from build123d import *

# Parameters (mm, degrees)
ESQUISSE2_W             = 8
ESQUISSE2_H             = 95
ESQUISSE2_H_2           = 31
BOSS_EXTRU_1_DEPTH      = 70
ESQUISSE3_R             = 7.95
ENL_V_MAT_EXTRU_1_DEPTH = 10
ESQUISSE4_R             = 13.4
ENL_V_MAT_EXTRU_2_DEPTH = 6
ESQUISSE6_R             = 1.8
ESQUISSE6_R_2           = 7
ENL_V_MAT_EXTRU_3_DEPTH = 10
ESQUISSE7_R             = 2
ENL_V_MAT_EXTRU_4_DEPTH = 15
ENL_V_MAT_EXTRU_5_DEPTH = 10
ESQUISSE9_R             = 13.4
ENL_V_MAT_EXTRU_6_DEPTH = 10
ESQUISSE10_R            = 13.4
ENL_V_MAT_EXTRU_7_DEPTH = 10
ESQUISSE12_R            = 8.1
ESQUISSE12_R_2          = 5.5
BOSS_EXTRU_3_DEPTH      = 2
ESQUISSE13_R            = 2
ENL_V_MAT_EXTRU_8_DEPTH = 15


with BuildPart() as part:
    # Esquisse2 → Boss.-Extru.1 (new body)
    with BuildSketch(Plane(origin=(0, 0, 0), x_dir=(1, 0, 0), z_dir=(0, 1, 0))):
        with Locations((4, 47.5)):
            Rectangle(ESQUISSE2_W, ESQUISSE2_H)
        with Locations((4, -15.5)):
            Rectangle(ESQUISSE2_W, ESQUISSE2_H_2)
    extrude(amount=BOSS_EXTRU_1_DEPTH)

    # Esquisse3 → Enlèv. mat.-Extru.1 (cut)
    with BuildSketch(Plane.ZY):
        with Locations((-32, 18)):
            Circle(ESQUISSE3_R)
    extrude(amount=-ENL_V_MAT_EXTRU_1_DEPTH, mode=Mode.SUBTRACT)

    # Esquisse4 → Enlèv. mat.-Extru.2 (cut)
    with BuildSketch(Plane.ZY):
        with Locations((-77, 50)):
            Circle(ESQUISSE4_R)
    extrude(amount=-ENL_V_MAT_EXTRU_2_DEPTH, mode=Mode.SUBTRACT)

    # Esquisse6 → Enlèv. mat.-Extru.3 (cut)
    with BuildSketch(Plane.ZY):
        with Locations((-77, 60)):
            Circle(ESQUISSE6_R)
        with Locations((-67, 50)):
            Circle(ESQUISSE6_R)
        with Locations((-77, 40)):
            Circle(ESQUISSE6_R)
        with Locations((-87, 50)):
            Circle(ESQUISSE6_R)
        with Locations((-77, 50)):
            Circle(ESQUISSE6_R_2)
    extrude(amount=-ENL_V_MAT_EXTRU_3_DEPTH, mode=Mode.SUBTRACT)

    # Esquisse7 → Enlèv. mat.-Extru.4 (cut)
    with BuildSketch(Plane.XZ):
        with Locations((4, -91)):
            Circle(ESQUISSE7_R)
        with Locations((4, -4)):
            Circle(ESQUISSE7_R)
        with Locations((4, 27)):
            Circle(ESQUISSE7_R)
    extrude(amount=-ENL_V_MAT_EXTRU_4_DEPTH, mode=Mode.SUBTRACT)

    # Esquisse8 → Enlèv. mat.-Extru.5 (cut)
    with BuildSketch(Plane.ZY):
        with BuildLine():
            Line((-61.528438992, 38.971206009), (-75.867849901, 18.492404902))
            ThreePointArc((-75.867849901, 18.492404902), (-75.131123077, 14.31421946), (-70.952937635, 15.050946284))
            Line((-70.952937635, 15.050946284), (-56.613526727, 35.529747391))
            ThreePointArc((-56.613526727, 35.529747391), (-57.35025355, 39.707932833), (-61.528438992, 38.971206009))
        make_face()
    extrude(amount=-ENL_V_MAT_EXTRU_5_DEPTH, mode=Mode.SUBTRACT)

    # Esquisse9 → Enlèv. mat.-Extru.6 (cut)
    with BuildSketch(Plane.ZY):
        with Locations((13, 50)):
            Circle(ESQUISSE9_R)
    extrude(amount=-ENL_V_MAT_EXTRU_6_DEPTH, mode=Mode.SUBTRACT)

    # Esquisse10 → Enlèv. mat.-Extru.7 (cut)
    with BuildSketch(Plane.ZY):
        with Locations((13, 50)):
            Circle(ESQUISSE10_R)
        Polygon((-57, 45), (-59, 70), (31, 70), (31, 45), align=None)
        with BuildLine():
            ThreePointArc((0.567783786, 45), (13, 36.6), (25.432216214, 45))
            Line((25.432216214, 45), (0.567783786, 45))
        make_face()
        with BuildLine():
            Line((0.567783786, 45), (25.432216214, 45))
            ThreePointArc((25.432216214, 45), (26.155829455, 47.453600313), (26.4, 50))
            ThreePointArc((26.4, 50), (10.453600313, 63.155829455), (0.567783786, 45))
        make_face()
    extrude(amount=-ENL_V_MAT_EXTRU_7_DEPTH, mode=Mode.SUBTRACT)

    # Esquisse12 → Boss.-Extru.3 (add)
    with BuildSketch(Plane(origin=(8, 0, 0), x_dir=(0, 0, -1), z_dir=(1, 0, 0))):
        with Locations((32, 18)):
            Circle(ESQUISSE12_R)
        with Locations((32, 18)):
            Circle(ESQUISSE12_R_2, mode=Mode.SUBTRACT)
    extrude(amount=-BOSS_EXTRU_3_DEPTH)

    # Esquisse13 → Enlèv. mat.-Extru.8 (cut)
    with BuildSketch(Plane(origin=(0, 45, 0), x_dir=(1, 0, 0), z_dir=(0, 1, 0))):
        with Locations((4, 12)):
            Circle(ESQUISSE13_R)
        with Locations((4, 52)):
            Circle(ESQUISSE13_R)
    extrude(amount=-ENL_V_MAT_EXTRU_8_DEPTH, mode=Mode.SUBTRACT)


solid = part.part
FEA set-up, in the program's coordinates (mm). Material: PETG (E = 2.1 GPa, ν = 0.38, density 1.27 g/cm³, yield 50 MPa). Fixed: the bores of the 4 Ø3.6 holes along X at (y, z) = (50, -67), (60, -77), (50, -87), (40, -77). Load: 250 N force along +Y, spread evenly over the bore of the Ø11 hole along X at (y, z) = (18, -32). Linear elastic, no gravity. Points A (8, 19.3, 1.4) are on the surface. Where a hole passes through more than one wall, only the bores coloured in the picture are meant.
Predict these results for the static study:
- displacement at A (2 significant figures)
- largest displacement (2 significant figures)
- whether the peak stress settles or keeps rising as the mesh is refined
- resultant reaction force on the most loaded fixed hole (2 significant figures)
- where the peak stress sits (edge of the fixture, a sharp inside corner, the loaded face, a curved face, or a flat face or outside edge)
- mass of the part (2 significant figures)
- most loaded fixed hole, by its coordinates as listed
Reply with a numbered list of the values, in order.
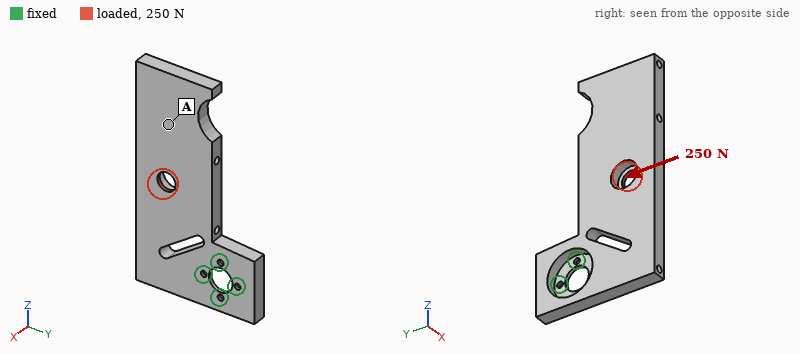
1. 0.79 mm
2. 1.1 mm
3. keeps rising
4. 390 N
5. edge of the fixture
6. 56 g
7. (50, -67)
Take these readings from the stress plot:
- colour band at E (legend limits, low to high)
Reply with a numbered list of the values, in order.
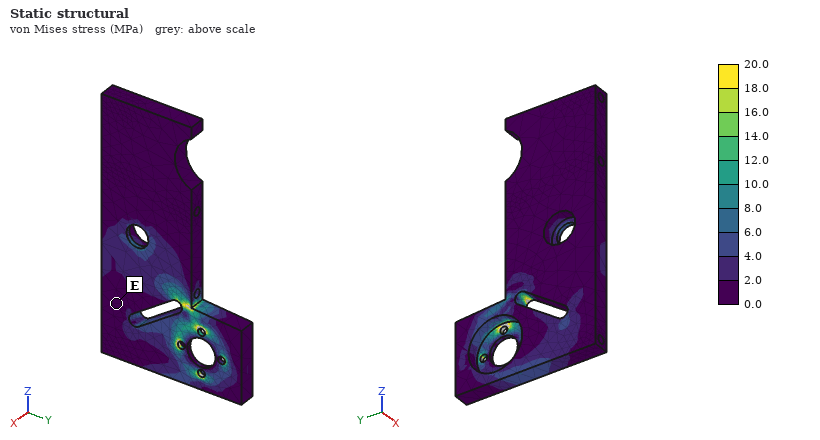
1. 0.0 to 2.0 MPa
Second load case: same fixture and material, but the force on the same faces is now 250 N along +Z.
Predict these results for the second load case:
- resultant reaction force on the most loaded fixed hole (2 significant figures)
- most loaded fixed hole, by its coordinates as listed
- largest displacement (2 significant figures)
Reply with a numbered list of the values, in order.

1. 260 N
2. (40, -77)
3. 1.6 mm
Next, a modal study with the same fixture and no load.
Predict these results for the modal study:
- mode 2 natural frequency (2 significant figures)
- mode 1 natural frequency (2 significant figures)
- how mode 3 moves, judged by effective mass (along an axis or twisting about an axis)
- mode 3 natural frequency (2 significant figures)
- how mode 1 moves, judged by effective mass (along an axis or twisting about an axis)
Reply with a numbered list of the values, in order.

1. 350 Hz
2. 90 Hz
3. along Y
4. 380 Hz
5. along X
